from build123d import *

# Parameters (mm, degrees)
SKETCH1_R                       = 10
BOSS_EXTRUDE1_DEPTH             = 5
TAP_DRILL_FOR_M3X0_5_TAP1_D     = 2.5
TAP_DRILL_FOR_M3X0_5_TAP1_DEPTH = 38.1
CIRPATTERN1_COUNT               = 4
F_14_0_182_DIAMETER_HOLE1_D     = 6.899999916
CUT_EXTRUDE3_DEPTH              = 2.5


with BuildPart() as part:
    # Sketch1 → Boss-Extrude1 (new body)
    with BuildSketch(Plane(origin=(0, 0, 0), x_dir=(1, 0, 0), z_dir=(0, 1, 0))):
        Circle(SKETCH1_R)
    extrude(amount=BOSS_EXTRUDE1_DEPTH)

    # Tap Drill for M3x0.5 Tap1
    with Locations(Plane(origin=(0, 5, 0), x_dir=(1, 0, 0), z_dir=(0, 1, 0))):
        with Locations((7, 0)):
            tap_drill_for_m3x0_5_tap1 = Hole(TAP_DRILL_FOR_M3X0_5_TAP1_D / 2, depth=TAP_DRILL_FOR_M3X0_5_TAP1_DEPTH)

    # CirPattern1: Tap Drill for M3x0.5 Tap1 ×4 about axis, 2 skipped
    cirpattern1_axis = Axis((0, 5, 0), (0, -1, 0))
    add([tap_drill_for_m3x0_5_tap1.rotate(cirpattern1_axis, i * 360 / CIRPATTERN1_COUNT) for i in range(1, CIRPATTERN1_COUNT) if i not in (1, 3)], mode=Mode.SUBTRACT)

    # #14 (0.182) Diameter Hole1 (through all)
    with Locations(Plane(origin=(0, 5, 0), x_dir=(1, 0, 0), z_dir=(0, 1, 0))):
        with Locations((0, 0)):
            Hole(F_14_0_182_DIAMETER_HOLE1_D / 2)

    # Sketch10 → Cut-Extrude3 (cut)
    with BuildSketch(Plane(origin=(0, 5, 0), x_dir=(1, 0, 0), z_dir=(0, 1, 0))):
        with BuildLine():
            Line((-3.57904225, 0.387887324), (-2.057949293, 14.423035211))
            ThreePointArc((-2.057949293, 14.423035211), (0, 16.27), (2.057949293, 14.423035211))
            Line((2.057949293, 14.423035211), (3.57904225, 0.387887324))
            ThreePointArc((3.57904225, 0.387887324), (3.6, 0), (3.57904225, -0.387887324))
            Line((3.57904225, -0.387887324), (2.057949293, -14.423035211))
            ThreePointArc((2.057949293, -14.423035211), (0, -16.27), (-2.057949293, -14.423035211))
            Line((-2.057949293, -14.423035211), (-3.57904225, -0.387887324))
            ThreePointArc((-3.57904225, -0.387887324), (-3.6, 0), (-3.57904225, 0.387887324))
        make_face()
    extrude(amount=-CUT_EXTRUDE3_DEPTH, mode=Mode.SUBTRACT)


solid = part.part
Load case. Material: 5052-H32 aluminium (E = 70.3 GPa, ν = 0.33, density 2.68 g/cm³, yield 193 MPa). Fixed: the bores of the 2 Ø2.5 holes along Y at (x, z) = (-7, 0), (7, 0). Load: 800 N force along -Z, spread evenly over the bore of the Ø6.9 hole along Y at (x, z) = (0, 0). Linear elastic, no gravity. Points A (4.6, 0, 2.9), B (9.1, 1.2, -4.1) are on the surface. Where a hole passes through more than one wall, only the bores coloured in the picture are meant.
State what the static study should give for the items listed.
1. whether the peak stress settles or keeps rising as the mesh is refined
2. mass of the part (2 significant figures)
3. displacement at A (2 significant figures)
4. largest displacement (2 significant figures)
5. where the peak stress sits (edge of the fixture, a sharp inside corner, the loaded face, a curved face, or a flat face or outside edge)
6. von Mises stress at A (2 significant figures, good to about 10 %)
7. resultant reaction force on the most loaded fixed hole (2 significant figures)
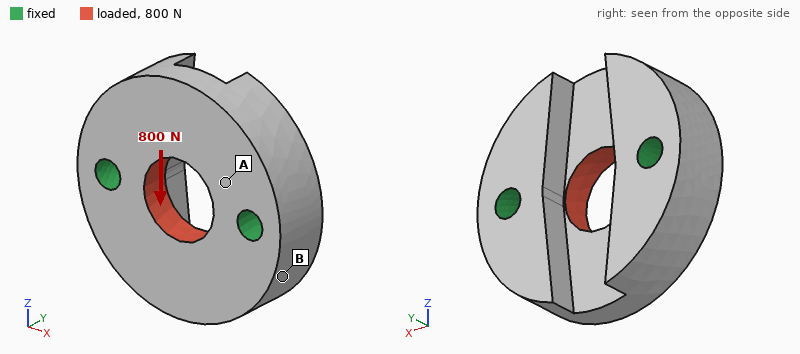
keeps rising
3.0 g
1.3 µm
3.4 µm
edge of the fixture
19 MPa
400 N
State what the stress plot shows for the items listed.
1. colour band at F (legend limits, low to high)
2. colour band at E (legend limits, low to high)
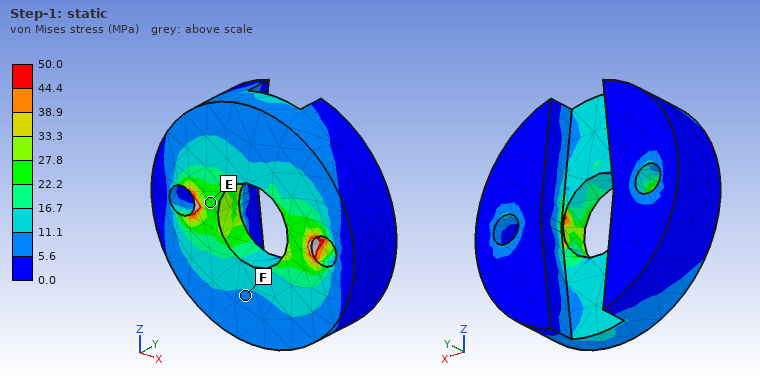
5.6 to 11.1 MPa
22.2 to 27.8 MPa
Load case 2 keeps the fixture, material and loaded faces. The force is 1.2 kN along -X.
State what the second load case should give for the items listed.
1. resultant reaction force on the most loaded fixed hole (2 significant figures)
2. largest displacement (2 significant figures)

600 N
2.9 µm
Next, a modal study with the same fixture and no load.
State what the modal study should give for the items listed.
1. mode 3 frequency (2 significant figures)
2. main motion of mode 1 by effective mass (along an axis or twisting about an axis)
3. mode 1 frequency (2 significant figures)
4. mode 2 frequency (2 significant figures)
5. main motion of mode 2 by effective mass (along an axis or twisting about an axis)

60 kHz
twisting about X
39 kHz
43 kHz
along Y
